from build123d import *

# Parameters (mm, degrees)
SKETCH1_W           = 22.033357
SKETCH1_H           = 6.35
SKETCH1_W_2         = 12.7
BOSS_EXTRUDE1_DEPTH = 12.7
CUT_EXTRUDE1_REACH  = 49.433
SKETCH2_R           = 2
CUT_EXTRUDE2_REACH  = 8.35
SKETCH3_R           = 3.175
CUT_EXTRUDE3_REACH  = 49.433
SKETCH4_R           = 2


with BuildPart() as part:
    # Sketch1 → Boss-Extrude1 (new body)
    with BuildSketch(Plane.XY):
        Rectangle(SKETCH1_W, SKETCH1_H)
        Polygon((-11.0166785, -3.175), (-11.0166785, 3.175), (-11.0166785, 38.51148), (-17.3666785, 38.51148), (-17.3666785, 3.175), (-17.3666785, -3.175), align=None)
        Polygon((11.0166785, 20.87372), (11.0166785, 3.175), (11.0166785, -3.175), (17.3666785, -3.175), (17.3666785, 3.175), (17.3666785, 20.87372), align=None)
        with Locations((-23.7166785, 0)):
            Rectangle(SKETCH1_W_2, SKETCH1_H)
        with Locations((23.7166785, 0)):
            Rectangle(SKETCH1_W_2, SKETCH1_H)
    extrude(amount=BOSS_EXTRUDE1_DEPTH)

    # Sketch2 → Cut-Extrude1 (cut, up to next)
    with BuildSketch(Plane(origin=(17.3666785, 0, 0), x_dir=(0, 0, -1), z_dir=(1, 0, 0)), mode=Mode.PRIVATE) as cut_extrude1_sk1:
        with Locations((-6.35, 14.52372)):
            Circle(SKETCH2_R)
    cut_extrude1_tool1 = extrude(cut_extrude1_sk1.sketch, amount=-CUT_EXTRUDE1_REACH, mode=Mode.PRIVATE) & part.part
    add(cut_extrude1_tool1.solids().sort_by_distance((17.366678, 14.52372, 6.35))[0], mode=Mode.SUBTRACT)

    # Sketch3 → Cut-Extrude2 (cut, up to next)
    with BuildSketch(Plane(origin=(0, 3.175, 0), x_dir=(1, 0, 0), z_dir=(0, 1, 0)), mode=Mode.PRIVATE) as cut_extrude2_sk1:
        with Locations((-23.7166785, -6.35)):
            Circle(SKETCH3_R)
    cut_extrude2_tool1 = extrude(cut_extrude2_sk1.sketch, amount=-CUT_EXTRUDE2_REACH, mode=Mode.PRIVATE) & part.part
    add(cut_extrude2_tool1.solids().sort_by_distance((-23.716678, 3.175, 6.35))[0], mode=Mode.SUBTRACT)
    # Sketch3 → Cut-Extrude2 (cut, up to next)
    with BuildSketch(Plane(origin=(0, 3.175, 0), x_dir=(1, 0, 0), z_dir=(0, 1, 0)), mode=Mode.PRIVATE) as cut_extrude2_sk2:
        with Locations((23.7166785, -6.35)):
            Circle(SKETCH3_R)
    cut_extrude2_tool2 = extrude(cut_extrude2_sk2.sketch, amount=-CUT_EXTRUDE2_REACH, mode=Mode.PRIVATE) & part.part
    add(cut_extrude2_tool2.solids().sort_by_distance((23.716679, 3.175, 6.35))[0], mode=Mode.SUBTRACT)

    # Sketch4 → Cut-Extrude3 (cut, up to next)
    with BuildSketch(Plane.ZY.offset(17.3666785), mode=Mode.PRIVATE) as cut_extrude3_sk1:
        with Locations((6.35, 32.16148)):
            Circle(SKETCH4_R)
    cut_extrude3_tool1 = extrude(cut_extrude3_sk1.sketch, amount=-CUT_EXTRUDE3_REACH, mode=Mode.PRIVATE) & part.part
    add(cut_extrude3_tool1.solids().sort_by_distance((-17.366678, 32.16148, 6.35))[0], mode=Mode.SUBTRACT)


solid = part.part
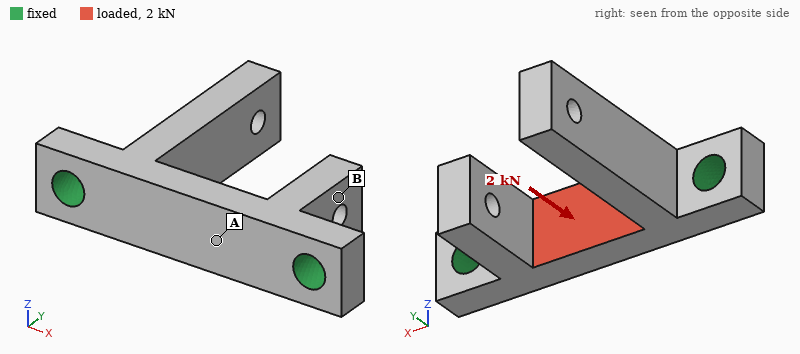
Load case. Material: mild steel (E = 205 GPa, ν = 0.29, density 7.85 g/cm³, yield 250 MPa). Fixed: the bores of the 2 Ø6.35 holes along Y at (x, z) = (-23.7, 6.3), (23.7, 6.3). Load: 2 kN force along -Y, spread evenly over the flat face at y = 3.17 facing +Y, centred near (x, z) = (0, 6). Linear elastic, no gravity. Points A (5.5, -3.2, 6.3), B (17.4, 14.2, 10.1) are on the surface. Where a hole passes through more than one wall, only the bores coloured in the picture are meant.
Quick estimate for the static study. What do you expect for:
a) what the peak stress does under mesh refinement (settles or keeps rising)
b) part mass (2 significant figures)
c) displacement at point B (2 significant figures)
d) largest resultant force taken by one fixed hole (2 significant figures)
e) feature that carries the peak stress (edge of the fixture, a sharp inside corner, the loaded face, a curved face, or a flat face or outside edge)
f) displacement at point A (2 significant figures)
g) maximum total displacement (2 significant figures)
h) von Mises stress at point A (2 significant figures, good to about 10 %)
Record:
keeps rising
67 g
13 µm
1.0 kN
edge of the fixture
13 µm
36 µm
55 MPa
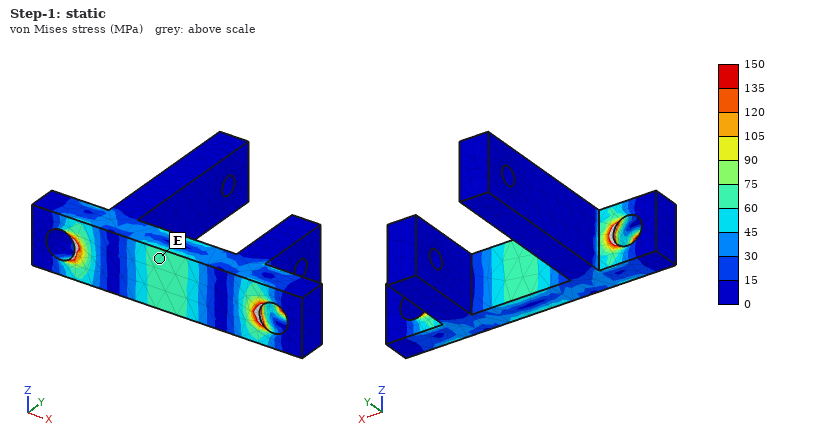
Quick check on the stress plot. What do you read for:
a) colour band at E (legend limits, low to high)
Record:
60 to 75 MPa
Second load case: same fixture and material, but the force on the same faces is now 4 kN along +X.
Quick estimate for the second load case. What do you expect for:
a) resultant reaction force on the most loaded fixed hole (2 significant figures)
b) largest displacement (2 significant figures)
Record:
2.0 kN
2.9 µm
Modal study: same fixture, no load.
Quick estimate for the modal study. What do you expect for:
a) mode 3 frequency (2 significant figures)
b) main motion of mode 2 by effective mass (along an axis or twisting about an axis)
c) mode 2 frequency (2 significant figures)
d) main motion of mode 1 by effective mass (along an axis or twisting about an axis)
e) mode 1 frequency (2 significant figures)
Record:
9700 Hz
along Z
4400 Hz
along X
3300 Hz
